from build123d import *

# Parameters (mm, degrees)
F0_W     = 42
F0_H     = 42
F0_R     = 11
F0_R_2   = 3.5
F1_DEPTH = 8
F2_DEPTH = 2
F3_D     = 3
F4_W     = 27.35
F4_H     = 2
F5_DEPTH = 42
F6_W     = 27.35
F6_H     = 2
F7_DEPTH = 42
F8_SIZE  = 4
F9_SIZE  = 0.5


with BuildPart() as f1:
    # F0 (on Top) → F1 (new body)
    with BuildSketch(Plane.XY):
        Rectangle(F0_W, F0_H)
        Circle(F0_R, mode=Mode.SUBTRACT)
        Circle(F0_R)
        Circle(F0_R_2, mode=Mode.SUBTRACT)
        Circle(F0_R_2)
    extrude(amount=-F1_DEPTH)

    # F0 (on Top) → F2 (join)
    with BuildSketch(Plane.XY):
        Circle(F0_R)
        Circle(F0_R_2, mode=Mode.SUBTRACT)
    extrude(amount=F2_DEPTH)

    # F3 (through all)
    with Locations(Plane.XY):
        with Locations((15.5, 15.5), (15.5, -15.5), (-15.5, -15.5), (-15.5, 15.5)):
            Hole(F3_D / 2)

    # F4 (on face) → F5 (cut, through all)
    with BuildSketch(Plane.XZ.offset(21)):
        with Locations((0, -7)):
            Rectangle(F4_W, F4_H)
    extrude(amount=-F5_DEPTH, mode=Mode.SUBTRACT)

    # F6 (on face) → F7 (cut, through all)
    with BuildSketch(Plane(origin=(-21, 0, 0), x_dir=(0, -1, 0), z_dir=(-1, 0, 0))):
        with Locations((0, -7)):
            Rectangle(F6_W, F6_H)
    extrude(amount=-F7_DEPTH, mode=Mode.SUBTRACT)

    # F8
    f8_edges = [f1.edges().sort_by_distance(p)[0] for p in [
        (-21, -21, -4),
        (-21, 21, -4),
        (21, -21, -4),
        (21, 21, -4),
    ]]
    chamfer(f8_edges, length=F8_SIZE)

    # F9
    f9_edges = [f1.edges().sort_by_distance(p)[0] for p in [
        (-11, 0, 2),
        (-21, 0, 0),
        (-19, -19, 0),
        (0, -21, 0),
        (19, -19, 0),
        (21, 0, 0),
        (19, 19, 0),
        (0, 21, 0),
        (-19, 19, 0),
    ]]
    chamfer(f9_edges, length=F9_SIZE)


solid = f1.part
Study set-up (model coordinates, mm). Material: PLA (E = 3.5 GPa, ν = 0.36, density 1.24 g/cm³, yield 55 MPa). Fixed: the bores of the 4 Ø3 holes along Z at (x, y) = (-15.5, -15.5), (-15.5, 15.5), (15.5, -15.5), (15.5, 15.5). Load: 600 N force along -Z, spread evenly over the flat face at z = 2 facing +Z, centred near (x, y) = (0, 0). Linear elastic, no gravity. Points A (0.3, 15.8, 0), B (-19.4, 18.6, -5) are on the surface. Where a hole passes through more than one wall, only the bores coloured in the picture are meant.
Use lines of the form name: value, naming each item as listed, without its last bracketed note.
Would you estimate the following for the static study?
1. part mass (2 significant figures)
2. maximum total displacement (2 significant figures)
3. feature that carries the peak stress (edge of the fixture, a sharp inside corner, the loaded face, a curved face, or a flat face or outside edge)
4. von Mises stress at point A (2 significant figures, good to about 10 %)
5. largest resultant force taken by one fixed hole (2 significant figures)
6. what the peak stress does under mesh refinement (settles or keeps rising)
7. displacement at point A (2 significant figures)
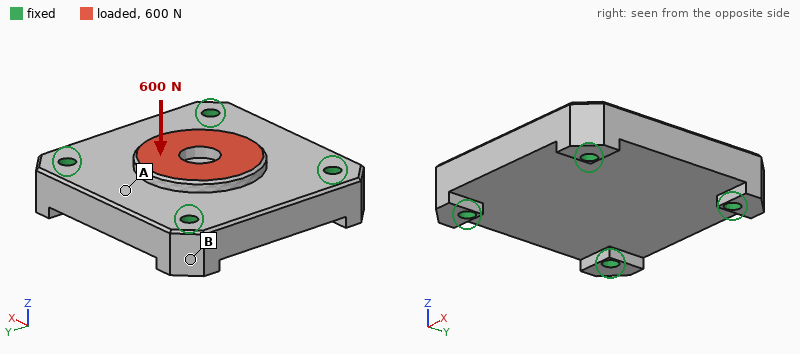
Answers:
part mass: 14 g
maximum total displacement: 73 µm
feature that carries the peak stress: edge of the fixture
von Mises stress at point A: 3.7 MPa
largest resultant force taken by one fixed hole: 160 N
what the peak stress does under mesh refinement: keeps rising
displacement at point A: 34 µm
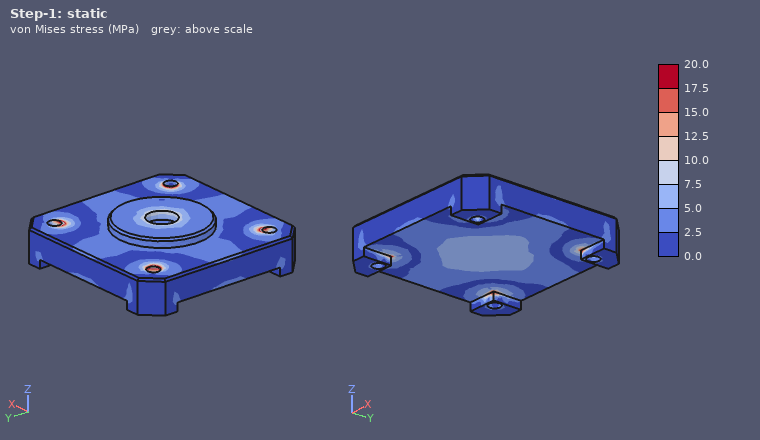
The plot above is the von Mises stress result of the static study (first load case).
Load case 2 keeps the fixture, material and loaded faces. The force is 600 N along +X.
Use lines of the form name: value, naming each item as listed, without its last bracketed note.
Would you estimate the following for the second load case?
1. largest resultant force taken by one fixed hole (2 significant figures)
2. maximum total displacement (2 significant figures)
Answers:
largest resultant force taken by one fixed hole: 170 N
maximum total displacement: 28 µm
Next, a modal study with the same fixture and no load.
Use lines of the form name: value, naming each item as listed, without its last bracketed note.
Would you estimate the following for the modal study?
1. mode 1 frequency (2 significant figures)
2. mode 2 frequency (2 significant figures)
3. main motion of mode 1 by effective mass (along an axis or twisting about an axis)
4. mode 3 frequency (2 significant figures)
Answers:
mode 1 frequency: 6400 Hz
mode 2 frequency: 9600 Hz
main motion of mode 1 by effective mass: along Z
mode 3 frequency: 9600 Hz
